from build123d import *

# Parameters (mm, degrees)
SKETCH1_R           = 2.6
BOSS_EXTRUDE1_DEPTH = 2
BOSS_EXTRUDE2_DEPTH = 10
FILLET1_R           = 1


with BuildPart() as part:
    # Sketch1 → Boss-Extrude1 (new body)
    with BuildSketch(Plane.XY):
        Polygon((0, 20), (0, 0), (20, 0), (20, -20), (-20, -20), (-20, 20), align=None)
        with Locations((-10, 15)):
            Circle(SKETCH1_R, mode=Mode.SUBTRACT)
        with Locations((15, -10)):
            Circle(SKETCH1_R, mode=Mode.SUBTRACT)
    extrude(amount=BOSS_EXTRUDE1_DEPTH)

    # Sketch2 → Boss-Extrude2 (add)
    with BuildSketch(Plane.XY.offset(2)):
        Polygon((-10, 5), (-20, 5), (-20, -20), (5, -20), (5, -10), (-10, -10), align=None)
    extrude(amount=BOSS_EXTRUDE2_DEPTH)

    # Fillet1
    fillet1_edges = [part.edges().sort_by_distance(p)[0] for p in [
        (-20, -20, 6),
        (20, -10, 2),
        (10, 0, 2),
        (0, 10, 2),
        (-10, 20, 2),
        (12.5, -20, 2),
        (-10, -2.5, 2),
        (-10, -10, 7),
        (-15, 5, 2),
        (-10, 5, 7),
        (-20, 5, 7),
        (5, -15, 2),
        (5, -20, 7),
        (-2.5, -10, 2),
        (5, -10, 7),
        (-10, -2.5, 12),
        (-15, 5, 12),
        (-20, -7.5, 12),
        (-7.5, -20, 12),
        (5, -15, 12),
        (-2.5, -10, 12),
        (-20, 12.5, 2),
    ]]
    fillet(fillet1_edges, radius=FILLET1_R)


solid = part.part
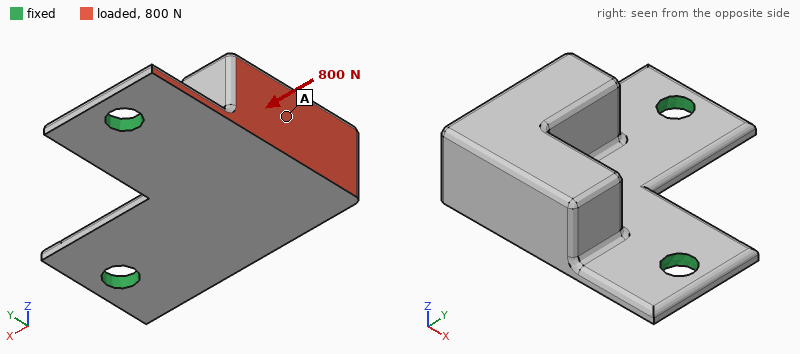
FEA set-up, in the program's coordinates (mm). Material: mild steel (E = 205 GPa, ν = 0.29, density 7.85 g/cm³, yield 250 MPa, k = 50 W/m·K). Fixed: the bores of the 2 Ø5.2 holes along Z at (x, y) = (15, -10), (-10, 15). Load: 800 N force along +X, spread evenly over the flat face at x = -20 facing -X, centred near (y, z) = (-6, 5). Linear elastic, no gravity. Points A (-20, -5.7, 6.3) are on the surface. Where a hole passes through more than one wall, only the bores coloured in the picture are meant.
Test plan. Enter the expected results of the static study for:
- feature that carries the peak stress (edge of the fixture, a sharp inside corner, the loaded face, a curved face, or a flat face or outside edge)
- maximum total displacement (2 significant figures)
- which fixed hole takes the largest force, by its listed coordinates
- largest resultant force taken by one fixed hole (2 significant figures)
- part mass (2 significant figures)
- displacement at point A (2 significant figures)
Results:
a curved face
0.10 mm
(15, -10)
600 N
49 g
0.065 mm
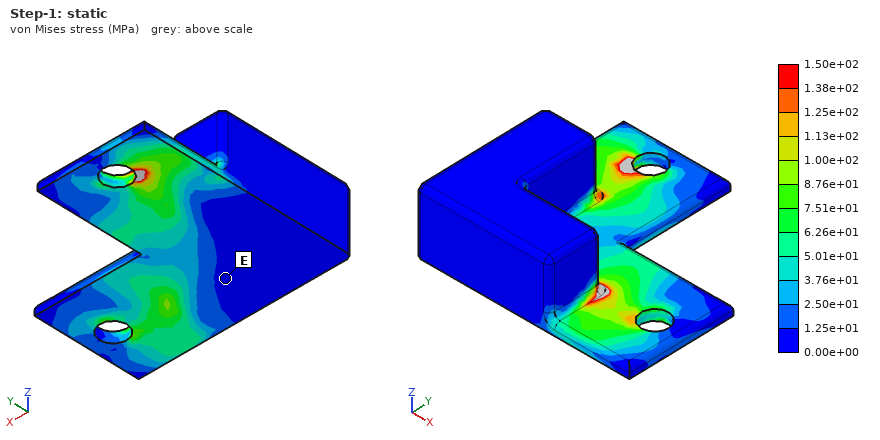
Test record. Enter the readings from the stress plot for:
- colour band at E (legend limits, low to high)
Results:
0.00e+00 to 1.25e+01 MPa
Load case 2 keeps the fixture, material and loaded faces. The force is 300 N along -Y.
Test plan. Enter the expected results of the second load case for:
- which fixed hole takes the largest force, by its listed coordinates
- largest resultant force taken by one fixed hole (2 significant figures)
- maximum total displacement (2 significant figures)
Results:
(-10, 15)
320 N
38 µm
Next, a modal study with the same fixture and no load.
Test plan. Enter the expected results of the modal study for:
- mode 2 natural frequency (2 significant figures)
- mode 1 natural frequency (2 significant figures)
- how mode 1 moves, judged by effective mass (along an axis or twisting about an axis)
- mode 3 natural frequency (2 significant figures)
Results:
7300 Hz
1400 Hz
along Z
9200 Hz
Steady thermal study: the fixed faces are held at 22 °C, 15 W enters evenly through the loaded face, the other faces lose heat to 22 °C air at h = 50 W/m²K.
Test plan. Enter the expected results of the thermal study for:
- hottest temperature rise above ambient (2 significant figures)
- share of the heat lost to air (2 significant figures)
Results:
52 K
30 %
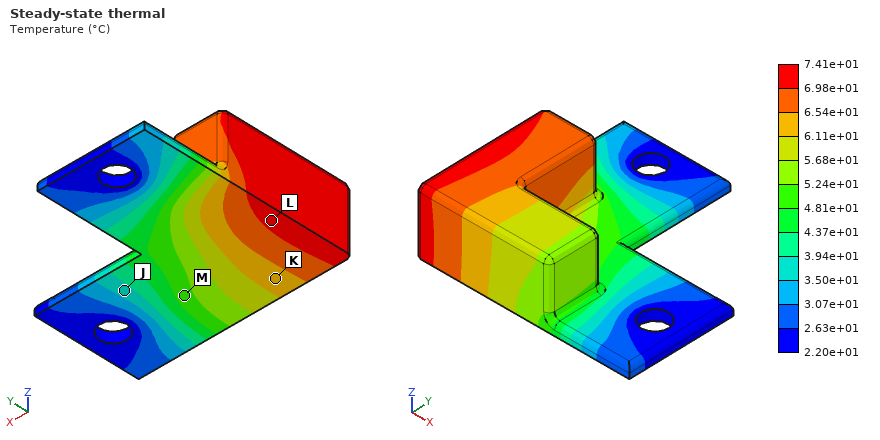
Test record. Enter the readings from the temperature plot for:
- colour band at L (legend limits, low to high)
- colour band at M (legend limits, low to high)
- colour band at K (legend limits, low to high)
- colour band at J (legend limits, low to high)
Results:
6.98e+01 to 7.41e+01 °C
4.81e+01 to 5.24e+01 °C
6.11e+01 to 6.54e+01 °C
3.50e+01 to 3.94e+01 °C
